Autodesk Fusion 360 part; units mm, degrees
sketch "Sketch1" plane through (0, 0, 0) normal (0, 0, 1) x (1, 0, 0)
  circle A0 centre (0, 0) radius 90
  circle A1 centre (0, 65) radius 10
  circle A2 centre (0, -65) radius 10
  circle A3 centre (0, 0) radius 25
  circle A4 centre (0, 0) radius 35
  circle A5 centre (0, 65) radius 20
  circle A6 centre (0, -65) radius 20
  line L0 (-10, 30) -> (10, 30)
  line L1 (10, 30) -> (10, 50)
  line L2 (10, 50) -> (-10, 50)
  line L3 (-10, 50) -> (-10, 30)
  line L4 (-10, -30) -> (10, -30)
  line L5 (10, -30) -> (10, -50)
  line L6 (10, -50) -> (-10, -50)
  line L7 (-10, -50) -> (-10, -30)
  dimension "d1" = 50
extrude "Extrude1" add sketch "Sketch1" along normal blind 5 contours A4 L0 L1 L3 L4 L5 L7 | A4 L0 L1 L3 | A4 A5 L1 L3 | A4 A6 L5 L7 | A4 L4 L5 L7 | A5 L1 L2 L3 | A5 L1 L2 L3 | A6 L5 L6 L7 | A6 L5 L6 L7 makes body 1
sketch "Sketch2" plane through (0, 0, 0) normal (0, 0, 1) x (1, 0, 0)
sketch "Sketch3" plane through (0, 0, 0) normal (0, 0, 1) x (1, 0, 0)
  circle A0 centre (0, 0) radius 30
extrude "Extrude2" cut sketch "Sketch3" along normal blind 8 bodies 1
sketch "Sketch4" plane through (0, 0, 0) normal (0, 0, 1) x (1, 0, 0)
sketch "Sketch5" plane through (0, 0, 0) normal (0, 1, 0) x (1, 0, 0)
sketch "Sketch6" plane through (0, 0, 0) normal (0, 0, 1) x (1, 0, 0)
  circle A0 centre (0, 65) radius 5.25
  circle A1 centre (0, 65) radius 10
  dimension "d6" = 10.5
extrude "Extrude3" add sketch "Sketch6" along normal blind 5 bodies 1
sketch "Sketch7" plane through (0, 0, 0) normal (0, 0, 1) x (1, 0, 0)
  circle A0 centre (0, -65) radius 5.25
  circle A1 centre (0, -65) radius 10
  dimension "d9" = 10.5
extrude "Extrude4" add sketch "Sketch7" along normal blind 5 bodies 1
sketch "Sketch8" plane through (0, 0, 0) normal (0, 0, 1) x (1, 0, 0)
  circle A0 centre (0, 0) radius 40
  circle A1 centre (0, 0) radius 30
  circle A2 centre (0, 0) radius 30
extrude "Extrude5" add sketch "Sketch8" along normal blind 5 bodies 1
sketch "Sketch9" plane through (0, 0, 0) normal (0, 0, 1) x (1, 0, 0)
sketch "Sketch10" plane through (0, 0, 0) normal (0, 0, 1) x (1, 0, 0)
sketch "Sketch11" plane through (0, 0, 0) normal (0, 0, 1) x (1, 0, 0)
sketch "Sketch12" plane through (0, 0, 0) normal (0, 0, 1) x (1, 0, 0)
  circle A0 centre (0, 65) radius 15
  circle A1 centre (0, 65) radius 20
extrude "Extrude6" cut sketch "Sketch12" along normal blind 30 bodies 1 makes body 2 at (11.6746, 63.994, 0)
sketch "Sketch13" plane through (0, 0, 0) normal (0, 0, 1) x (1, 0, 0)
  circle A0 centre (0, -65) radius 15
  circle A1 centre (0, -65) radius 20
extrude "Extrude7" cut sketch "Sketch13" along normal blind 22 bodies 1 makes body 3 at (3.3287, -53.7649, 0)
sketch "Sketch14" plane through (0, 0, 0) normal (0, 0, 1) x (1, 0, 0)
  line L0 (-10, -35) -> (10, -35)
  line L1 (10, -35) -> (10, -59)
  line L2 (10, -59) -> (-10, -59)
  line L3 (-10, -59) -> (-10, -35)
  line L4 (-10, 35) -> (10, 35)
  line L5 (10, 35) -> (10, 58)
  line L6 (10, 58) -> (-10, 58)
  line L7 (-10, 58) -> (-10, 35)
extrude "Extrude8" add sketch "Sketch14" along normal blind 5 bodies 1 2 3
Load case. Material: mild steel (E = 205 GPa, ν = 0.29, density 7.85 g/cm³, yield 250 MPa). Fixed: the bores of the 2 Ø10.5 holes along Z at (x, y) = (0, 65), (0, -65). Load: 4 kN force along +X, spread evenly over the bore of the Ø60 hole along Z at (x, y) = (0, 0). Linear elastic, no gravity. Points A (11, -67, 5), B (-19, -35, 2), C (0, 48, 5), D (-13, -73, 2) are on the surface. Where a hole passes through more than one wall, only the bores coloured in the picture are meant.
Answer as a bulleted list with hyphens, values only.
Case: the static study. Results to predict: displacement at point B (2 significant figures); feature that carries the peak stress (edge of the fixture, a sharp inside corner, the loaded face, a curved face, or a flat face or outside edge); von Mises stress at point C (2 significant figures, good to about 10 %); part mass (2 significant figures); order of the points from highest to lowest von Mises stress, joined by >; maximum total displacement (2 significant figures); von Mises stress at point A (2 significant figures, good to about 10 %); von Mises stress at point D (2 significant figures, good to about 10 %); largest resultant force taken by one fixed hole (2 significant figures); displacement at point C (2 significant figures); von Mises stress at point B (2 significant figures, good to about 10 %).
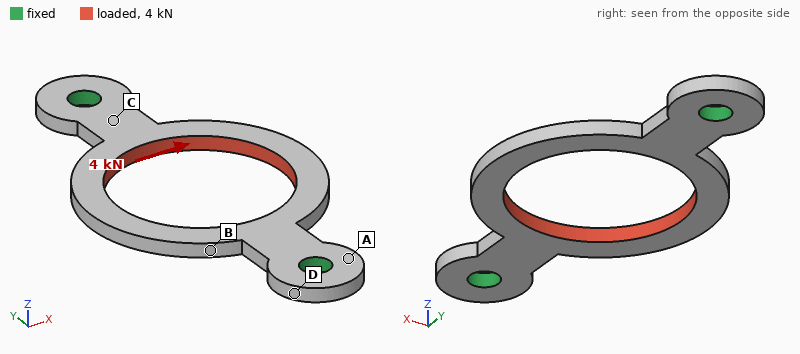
- 20 µm
- edge of the fixture
- 49 MPa
- 150 g
- C > B > A > D
- 21 µm
- 19 MPa
- 10 MPa
- 2.0 kN
- 8.2 µm
- 37 MPa
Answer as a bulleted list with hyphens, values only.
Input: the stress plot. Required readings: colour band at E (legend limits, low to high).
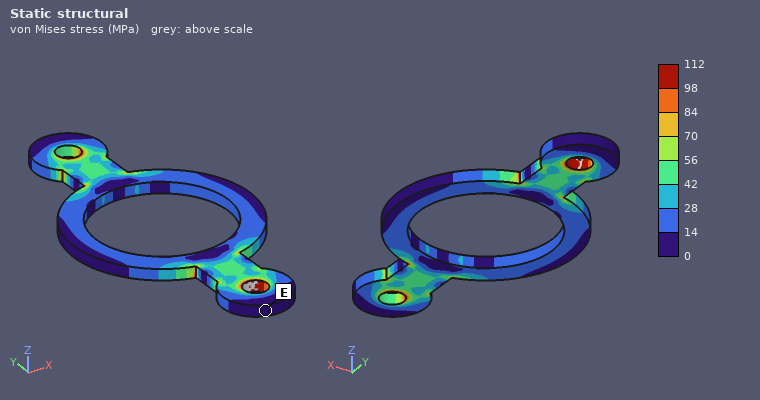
- 0 to 14 MPa
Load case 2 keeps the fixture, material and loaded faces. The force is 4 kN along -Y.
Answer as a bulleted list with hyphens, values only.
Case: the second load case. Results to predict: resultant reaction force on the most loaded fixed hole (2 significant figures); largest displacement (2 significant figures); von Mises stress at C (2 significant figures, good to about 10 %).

- 2.0 kN
- 17 µm
- 17 MPa
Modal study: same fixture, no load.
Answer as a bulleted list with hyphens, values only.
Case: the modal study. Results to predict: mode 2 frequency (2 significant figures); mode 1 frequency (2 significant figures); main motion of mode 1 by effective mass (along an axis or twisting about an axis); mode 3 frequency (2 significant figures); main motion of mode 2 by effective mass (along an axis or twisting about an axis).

- 1300 Hz
- 1200 Hz
- twisting about Y
- 3500 Hz
- along Z
